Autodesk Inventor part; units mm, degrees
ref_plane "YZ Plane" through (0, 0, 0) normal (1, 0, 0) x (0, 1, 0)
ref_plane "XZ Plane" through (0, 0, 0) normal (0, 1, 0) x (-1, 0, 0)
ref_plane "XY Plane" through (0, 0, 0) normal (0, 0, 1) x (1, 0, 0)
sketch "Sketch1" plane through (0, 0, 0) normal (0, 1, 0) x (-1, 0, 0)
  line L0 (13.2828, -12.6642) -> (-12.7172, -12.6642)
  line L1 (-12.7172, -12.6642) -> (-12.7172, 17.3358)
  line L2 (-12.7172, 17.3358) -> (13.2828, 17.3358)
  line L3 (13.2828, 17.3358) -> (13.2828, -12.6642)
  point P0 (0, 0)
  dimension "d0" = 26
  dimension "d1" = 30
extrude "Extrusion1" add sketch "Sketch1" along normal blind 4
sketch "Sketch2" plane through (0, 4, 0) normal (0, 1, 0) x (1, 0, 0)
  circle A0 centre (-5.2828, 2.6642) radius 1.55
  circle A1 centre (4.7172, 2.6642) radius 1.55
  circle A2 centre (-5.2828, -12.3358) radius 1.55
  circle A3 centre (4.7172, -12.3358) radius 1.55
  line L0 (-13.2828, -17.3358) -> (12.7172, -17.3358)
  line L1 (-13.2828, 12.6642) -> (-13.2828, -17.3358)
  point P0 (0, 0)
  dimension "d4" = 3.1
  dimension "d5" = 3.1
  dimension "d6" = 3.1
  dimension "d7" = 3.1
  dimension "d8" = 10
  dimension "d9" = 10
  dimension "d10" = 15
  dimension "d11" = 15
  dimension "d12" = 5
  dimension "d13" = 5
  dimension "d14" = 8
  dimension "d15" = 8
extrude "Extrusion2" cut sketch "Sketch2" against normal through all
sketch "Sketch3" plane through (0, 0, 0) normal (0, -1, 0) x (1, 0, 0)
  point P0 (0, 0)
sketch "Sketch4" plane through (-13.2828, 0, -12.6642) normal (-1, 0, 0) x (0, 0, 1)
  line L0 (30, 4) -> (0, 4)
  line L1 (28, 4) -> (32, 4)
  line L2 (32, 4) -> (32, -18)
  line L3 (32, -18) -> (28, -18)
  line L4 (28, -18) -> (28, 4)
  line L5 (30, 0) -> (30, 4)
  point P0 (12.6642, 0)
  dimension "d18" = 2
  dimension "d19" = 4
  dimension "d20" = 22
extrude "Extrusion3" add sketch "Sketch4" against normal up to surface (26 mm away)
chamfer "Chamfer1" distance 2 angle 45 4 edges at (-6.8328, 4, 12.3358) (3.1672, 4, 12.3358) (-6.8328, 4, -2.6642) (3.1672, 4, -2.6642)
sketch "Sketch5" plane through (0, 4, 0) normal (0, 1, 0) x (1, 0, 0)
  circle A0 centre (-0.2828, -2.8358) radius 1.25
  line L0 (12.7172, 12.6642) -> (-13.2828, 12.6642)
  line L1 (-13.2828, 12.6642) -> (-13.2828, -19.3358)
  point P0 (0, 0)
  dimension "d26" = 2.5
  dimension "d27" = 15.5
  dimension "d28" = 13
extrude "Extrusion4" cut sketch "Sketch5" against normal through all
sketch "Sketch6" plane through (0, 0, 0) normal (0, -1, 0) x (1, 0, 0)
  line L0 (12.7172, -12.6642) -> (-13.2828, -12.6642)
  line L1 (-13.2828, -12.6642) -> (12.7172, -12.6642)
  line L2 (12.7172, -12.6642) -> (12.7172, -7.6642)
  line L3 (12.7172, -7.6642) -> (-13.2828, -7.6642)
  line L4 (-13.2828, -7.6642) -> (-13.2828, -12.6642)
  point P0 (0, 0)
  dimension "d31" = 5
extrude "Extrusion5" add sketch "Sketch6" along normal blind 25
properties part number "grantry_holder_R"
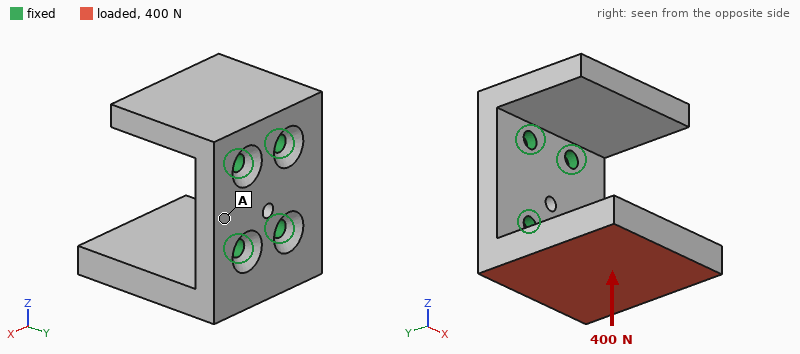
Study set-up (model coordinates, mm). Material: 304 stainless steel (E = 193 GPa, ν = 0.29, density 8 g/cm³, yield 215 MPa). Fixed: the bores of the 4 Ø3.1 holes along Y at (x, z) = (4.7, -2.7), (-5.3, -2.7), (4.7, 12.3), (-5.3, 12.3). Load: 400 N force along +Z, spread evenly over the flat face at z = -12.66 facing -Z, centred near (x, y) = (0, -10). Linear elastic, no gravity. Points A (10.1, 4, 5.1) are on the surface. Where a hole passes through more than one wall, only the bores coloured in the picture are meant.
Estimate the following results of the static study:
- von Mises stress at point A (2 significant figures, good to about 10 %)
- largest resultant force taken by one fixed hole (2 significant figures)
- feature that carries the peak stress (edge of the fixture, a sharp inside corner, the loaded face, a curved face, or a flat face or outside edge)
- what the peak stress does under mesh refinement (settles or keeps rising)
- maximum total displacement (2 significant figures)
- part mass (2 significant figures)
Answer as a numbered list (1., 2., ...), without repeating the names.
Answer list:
1. 14 MPa
2. 350 N
3. edge of the fixture
4. keeps rising
5. 62 µm
6. 66 g
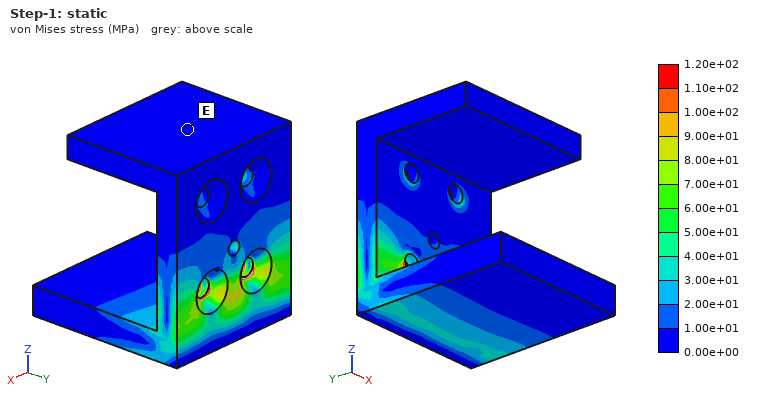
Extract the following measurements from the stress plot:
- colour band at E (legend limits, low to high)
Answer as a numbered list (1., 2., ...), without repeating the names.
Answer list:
1. 0.00e+00 to 1.00e+01 MPa
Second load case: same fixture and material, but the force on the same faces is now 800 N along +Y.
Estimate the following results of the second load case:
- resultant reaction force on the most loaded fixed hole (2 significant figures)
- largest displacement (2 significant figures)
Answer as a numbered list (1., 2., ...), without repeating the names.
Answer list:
1. 590 N
2. 67 µm
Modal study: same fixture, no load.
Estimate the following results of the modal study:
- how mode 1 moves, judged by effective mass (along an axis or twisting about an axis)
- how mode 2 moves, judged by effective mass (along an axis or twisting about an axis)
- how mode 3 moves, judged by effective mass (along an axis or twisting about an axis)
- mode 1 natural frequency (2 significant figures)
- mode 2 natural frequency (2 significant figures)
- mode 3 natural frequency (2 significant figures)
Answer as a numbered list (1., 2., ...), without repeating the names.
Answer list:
1. along Z
2. along Z
3. along X
4. 2800 Hz
5. 5200 Hz
6. 5500 Hz
